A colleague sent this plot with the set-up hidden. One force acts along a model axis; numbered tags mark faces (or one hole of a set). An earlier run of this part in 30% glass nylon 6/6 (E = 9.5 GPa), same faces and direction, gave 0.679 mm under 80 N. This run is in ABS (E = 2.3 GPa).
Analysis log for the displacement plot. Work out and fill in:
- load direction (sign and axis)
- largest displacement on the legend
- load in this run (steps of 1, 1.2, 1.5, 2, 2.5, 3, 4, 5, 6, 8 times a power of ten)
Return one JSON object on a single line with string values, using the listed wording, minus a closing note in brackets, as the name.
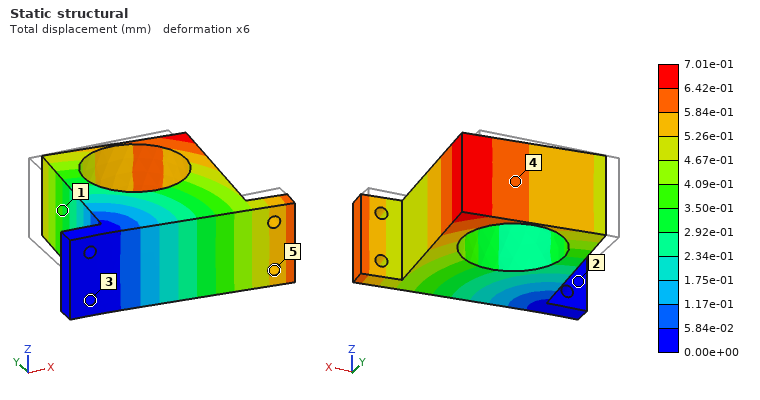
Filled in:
{"load direction": "-Y", "largest displacement on the legend": "7.01e-01 mm", "load in this run": "20 N"}
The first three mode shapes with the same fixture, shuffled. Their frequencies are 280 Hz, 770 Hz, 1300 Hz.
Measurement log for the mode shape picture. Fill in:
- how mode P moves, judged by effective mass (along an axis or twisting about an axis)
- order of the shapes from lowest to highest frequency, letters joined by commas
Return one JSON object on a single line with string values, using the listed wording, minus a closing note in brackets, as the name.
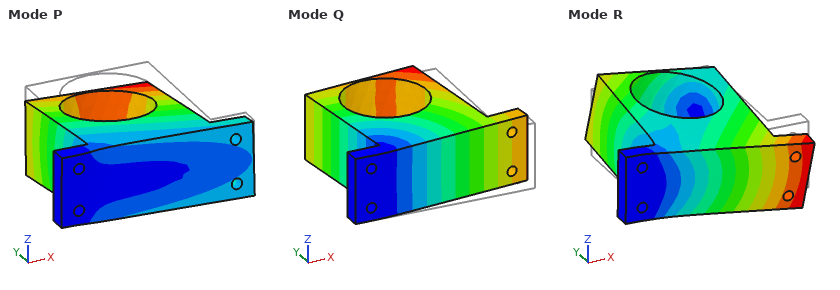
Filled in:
{"how mode P moves, judged by effective mass": "along Z", "order of the shapes from lowest to highest frequency, letters joined by commas": "Q, P, R"}
